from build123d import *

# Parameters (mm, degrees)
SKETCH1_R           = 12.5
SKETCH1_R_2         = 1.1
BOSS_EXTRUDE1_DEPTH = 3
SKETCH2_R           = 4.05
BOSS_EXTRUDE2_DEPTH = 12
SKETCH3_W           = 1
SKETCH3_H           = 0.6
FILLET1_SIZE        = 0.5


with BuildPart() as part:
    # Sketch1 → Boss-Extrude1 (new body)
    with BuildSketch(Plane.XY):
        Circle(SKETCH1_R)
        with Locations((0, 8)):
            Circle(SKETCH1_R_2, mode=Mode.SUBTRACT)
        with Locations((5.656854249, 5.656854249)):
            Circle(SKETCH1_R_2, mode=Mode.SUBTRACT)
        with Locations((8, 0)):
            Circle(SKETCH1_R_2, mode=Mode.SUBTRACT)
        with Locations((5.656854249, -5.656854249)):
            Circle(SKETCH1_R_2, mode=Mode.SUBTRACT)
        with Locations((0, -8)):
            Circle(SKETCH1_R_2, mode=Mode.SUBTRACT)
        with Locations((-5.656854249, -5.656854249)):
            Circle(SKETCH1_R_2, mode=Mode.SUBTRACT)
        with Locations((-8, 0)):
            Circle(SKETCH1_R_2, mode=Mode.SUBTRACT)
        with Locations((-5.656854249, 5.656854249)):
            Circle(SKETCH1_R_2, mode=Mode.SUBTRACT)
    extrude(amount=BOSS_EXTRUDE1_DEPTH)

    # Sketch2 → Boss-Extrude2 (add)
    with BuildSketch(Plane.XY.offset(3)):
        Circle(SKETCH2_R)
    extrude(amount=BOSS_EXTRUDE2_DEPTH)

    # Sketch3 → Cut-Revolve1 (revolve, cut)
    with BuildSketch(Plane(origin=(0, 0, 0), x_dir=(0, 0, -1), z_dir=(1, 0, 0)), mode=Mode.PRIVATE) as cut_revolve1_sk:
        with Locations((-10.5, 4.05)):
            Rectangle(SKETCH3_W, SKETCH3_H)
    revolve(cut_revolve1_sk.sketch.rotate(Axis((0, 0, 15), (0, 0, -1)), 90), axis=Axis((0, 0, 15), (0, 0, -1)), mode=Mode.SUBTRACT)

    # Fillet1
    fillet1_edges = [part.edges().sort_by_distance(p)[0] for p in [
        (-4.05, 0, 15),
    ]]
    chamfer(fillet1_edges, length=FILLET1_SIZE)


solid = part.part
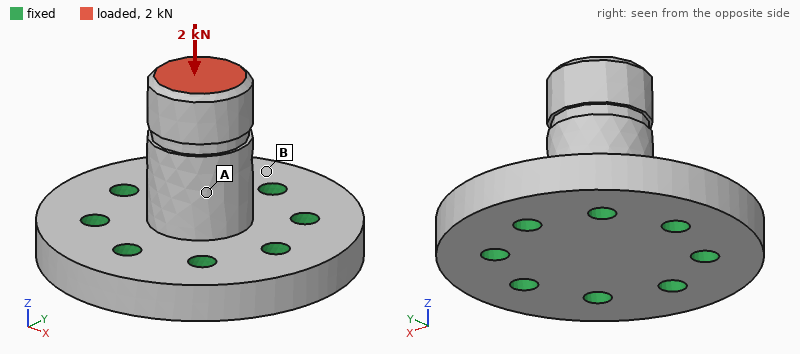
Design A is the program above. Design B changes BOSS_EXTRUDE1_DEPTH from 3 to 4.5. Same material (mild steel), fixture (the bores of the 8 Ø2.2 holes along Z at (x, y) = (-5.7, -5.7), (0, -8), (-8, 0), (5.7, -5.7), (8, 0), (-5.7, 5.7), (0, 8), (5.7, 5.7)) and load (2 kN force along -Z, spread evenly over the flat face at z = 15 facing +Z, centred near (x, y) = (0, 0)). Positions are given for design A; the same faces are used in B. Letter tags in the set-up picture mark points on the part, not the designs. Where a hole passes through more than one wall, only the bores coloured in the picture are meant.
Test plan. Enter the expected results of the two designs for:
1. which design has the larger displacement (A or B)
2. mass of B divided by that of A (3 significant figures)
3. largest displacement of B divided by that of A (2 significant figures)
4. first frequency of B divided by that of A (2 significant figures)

A
1.31
0.74
1.3
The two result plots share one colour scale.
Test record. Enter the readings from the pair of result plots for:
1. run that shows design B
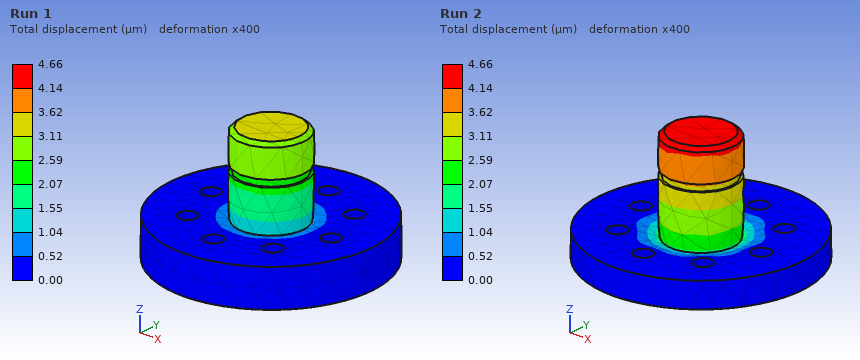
Run 1
